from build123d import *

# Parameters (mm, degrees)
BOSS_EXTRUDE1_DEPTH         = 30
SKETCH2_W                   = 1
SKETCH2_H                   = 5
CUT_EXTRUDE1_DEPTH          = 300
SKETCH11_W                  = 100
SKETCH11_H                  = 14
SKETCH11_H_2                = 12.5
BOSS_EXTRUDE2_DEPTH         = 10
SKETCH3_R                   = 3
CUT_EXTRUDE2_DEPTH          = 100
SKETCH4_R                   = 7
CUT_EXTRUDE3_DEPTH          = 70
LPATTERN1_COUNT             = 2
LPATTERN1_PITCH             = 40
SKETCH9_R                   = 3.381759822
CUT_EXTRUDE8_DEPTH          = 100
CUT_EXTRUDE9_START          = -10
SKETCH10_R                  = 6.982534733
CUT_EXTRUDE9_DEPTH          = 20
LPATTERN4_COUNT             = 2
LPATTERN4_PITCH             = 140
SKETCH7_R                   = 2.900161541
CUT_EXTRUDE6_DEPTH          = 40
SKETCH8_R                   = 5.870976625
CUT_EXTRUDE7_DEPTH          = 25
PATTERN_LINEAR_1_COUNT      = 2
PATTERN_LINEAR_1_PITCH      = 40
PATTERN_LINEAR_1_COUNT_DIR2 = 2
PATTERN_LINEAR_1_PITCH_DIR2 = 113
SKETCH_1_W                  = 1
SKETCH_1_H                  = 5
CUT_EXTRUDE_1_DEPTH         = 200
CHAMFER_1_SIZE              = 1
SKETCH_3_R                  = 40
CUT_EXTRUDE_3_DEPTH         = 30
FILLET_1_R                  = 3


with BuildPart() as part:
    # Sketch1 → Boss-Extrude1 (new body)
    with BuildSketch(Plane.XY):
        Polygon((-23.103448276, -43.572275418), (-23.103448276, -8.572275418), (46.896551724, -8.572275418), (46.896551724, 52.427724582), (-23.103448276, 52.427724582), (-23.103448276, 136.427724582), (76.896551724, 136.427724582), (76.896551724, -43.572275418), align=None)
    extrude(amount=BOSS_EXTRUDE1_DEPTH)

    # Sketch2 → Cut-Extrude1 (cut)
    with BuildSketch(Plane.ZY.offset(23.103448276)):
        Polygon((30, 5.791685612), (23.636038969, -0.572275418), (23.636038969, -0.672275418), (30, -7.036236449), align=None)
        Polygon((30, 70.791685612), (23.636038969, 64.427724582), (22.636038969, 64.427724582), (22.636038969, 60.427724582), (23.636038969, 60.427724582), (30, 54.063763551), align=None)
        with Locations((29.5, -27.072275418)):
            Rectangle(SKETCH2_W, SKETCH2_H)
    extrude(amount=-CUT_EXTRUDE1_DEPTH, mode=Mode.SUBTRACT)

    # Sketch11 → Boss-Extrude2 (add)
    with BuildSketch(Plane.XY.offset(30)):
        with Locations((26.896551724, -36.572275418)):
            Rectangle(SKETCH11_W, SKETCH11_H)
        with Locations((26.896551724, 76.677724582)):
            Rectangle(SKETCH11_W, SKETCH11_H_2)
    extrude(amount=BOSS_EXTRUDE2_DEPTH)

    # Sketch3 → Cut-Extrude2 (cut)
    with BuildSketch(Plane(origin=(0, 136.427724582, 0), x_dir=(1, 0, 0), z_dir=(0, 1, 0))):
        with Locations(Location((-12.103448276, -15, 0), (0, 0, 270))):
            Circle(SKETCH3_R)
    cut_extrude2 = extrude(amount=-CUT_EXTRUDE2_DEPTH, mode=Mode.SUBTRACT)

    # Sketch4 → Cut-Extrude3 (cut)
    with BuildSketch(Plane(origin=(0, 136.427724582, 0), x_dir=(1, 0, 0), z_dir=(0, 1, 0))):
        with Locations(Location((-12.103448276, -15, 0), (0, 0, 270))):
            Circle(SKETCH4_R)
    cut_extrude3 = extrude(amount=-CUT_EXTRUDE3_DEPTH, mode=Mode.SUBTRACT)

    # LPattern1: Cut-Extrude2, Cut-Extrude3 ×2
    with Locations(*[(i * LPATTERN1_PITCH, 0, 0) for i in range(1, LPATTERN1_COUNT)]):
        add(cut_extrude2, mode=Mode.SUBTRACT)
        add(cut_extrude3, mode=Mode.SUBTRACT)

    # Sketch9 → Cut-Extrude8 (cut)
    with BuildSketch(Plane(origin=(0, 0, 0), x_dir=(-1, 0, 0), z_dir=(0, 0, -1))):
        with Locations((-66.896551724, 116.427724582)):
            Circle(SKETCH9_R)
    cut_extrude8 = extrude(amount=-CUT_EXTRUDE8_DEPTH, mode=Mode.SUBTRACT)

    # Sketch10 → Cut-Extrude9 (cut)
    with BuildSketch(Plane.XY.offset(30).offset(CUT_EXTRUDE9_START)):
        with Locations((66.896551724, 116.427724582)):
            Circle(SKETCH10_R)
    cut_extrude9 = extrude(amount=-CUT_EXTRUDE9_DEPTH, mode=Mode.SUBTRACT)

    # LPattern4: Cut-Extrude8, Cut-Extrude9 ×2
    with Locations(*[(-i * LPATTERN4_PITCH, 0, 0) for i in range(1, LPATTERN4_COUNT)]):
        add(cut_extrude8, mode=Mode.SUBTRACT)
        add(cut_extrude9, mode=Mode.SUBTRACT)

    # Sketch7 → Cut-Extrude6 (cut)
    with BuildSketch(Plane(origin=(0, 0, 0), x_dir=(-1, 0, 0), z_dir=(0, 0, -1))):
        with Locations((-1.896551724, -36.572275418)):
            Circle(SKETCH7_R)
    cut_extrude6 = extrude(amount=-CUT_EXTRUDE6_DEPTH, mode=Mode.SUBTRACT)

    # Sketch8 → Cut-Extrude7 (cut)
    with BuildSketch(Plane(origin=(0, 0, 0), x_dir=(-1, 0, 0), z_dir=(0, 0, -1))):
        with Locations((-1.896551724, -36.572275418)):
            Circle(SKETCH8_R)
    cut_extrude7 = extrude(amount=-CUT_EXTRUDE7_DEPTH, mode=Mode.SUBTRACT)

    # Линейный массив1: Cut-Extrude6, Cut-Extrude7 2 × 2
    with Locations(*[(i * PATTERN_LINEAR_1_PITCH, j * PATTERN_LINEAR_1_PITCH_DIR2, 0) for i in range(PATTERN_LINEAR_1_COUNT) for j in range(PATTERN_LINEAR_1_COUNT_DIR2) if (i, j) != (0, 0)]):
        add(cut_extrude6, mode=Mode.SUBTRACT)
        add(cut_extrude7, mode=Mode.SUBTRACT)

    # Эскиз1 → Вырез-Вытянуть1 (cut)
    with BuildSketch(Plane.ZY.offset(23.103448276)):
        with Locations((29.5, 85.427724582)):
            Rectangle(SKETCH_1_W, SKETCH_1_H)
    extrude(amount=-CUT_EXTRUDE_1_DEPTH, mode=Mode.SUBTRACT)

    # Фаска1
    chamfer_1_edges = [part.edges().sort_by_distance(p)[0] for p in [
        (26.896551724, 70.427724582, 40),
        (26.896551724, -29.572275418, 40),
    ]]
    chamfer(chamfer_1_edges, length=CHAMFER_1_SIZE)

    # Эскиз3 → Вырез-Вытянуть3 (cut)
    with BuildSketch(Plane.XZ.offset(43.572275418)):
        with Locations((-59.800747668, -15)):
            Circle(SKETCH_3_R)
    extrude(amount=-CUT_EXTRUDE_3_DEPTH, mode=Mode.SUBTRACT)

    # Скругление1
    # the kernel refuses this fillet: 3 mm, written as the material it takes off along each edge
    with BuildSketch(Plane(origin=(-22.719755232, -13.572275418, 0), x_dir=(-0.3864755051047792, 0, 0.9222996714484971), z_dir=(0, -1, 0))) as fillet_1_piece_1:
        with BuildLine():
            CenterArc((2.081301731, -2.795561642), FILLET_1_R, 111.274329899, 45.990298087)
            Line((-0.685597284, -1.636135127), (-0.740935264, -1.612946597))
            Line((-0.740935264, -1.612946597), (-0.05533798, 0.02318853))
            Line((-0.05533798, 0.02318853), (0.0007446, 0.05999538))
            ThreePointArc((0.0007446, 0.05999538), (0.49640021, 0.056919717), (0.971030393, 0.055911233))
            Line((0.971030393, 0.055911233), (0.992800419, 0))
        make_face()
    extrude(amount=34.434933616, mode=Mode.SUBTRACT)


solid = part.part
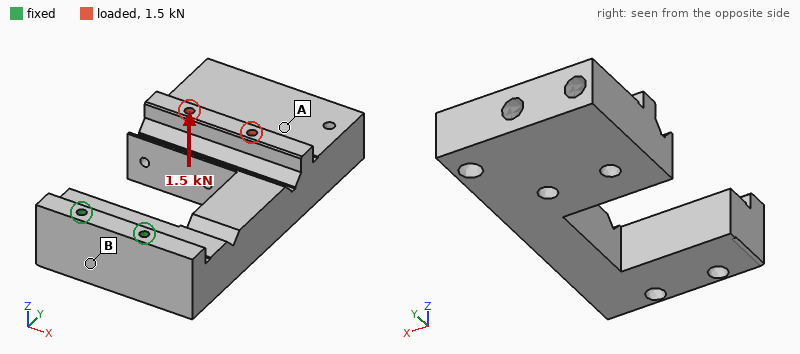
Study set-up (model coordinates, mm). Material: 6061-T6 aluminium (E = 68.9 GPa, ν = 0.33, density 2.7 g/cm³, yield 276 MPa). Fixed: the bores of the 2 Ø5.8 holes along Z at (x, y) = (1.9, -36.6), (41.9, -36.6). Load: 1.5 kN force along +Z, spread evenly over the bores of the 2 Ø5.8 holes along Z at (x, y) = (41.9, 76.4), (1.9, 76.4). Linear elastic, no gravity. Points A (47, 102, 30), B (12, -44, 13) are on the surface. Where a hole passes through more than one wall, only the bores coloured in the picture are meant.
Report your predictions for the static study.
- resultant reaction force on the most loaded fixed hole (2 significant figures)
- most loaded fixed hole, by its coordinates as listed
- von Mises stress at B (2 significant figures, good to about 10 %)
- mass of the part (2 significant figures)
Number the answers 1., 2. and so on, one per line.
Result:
1. 1.0 kN
2. (41.9, -36.6)
3. 16 MPa
4. 1.1 kg
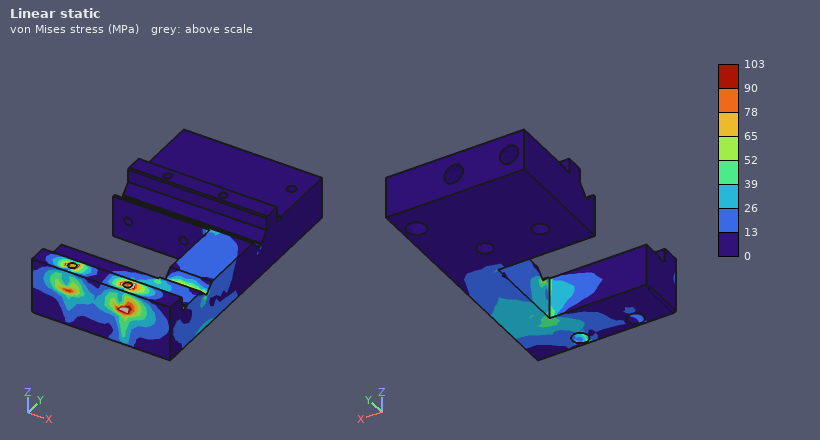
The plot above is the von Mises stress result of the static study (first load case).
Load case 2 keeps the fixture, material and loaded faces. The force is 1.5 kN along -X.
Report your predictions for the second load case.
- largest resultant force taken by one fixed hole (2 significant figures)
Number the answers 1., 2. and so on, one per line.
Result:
1. 4.0 kN
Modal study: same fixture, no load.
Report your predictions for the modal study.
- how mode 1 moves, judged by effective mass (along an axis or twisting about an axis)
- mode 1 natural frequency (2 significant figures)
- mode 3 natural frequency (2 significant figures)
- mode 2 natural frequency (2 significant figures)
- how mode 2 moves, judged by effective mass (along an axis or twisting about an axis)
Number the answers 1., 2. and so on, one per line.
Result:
1. along Z
2. 270 Hz
3. 1000 Hz
4. 390 Hz
5. along X
